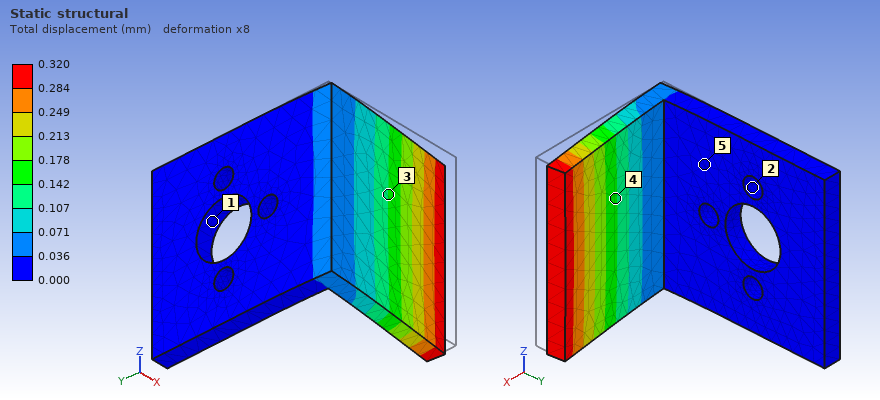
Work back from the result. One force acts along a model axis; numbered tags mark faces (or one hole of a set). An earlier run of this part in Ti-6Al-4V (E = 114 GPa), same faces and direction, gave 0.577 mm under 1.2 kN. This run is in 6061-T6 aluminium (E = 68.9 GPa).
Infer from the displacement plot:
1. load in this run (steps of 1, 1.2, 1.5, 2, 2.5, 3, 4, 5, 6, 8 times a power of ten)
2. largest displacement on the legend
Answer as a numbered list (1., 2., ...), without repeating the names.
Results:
1. 400 N
2. 0.320 mm
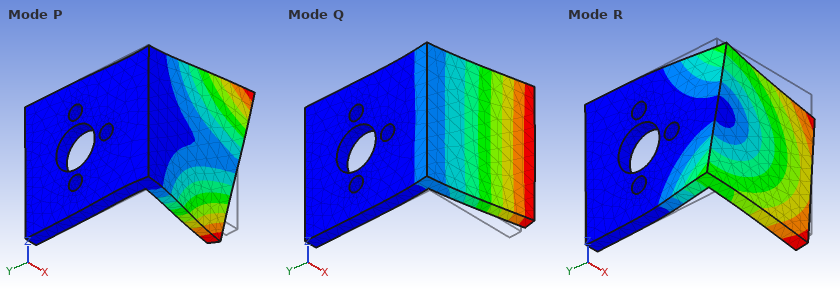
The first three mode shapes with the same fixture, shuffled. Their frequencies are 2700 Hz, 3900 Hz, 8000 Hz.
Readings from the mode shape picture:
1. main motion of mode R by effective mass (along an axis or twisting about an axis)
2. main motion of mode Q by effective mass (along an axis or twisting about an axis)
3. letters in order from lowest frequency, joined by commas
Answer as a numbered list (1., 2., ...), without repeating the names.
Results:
1. along Z
2. along Y
3. Q, R, P
